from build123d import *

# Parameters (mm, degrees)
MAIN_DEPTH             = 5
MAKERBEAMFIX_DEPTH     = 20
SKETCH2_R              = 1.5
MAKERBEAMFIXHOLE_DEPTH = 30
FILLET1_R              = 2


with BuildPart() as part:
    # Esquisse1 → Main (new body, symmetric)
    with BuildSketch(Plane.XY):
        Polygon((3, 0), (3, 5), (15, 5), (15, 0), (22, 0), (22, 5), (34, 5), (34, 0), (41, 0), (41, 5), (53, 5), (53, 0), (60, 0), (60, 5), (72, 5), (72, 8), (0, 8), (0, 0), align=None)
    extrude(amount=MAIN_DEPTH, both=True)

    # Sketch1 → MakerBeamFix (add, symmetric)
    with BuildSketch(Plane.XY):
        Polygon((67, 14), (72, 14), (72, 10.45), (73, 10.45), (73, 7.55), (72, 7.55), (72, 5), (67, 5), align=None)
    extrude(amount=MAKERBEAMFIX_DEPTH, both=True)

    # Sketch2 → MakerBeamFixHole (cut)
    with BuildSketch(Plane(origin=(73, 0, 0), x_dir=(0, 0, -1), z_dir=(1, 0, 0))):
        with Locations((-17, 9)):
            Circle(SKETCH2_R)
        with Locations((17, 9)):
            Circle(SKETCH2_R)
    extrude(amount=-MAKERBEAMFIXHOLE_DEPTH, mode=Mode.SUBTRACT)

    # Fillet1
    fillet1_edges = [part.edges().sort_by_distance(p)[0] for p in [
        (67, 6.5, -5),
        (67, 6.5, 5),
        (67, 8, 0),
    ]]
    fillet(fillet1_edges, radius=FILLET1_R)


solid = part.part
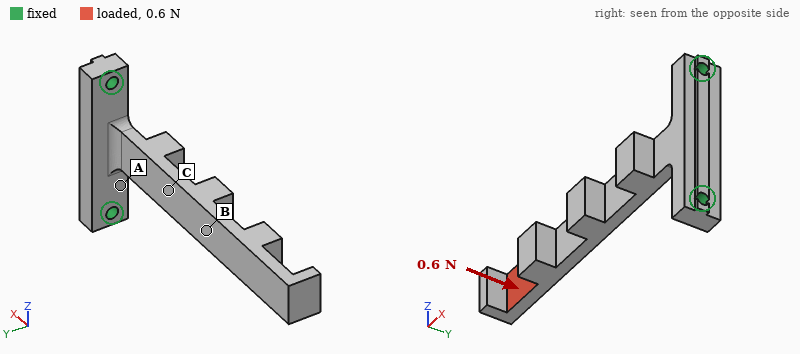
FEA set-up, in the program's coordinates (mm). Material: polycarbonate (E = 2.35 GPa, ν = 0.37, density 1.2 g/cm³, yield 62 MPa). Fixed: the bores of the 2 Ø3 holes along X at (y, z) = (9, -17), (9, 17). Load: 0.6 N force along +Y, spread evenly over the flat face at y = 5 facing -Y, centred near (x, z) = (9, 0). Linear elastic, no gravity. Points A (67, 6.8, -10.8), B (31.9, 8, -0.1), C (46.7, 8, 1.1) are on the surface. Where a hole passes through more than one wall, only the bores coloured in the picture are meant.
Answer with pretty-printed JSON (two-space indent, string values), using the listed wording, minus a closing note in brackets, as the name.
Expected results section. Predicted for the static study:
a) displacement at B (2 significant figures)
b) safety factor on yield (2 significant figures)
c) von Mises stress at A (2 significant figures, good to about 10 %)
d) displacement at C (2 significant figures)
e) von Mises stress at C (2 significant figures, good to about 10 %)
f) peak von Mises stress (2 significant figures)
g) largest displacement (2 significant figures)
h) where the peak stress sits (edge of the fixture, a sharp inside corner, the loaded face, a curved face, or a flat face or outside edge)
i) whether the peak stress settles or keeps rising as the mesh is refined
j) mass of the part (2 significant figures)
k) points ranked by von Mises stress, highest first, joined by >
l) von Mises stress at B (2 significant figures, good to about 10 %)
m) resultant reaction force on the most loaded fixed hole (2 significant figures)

{
  "displacement at B": "0.30 mm",
  "safety factor on yield": "20",
  "von Mises stress at A": "0.41 MPa",
  "displacement at C": "0.12 mm",
  "von Mises stress at C": "1.4 MPa",
  "peak von Mises stress": "3.0 MPa",
  "largest displacement": "0.79 mm",
  "where the peak stress sits": "a curved face",
  "whether the peak stress settles or keeps rising as the mesh is refined": "settles",
  "mass of the part": "6.1 g",
  "points ranked by von Mises stress, highest first, joined by >": "C > B > A",
  "von Mises stress at B": "0.82 MPa",
  "resultant reaction force on the most loaded fixed hole": "0.42 N"
}
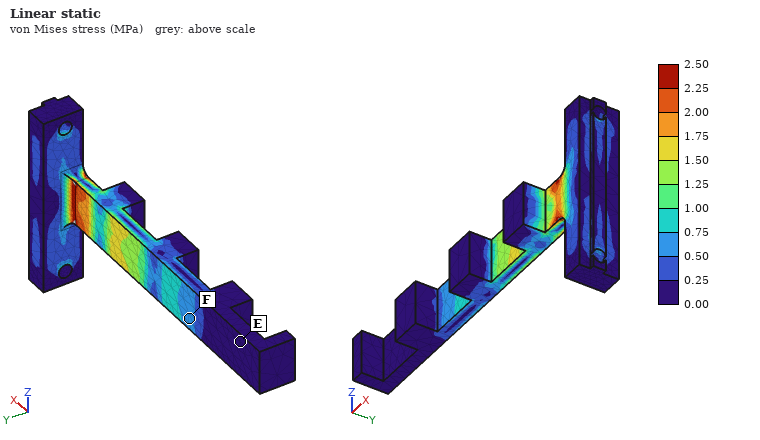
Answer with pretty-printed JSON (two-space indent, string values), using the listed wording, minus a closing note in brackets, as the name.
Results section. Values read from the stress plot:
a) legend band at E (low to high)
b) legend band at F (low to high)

{
  "legend band at E": "0.00 to 0.25 MPa",
  "legend band at F": "0.50 to 0.75 MPa"
}
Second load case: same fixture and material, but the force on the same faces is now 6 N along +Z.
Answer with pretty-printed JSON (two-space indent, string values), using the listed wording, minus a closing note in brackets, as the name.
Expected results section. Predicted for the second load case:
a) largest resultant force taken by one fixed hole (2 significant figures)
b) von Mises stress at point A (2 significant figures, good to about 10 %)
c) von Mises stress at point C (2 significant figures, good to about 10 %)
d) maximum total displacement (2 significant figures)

{
  "largest resultant force taken by one fixed hole": "16 N",
  "von Mises stress at point A": "0.81 MPa",
  "von Mises stress at point C": "0.94 MPa",
  "maximum total displacement": "0.96 mm"
}
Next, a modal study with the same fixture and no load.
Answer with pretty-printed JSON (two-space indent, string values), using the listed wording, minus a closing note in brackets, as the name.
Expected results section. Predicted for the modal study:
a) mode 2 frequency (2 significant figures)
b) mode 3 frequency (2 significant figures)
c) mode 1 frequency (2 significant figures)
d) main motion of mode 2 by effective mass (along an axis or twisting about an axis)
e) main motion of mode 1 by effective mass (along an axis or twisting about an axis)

{
  "mode 2 frequency": "360 Hz",
  "mode 3 frequency": "750 Hz",
  "mode 1 frequency": "130 Hz",
  "main motion of mode 2 by effective mass": "along Z",
  "main motion of mode 1 by effective mass": "along Y"
}
